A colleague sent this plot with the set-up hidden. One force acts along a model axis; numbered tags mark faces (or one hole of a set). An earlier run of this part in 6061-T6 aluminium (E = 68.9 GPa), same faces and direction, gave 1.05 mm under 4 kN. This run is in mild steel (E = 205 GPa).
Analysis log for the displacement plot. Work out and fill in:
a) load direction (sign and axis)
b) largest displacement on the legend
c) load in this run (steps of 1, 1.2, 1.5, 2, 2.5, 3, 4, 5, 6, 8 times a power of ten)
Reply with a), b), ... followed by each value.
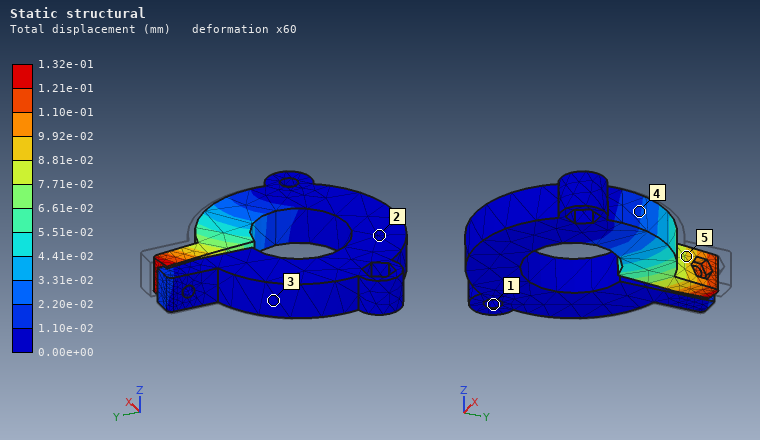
a) -X
b) 1.32e-01 mm
c) 1.5 kN
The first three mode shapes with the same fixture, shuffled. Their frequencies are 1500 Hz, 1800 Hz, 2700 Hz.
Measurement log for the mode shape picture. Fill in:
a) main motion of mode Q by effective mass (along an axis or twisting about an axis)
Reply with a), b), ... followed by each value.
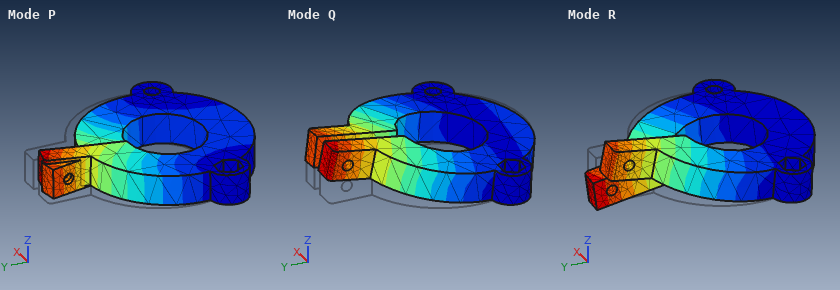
a) along Z
